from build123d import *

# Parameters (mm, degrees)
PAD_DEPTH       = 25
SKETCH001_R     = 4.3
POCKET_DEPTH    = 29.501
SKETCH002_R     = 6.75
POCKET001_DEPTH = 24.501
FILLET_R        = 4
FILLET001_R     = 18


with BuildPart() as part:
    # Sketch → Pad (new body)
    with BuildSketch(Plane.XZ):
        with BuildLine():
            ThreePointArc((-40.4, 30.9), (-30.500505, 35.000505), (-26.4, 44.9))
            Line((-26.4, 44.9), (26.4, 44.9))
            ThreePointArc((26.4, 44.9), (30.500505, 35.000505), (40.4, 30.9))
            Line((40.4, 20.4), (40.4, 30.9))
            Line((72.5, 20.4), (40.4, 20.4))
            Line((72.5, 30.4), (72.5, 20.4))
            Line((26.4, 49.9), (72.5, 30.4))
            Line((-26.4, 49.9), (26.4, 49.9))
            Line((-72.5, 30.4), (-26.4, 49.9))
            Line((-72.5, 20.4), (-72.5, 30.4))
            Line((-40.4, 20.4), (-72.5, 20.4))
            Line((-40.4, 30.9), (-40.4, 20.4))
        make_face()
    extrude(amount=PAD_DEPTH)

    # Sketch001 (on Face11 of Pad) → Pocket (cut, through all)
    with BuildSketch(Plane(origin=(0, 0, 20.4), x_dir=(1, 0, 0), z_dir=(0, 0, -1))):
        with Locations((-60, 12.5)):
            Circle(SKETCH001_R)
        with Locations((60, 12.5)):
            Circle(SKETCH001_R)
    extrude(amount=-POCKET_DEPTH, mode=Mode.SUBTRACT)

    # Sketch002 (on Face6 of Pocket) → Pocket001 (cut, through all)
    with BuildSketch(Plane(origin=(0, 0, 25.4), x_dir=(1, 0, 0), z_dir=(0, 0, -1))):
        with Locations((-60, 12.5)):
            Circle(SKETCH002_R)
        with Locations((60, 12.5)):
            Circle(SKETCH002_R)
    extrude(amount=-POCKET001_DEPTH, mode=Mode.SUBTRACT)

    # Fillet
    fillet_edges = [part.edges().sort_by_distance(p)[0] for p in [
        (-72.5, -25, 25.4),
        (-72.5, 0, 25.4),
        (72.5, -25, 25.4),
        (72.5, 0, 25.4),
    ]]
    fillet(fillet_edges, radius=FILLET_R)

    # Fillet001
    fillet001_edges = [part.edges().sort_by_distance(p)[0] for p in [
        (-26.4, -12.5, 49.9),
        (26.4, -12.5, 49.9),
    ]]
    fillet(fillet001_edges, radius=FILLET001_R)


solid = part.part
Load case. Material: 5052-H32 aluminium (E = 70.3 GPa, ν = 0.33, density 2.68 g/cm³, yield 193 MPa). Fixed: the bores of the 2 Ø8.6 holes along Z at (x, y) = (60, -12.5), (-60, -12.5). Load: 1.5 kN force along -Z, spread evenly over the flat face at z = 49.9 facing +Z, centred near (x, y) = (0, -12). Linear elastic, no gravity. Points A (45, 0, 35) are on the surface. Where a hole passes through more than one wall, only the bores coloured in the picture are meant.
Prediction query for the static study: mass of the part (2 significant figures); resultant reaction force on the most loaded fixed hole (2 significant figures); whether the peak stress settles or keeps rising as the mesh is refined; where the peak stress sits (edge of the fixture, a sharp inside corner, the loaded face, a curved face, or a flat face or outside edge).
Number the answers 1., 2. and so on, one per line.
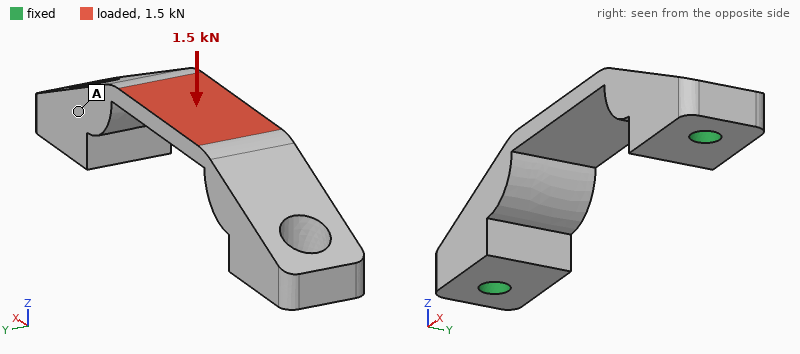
1. 100 g
2. 1.4 kN
3. keeps rising
4. a sharp inside corner
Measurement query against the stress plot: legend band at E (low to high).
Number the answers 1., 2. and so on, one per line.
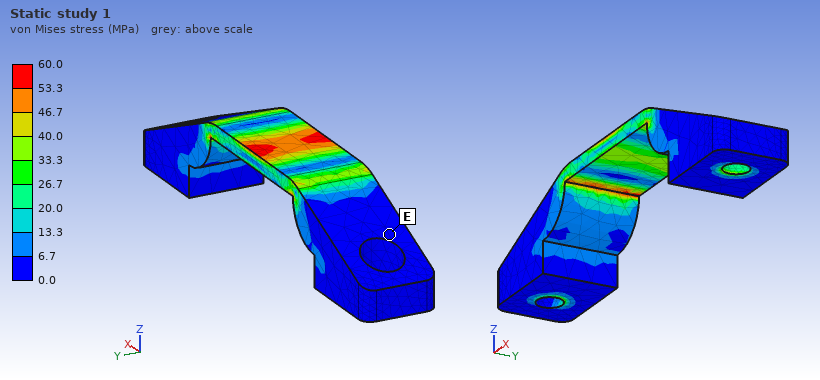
1. 0.0 to 6.7 MPa
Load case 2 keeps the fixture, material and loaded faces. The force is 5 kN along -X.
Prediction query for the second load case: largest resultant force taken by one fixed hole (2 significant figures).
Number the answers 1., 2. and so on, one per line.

1. 2.6 kN
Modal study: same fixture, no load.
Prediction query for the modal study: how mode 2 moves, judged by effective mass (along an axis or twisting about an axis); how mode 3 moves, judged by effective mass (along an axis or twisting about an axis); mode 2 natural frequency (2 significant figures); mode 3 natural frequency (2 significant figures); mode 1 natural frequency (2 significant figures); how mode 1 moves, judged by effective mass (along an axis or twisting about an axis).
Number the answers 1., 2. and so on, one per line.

1. along X
2. along Z
3. 4300 Hz
4. 6500 Hz
5. 4000 Hz
6. along Y
